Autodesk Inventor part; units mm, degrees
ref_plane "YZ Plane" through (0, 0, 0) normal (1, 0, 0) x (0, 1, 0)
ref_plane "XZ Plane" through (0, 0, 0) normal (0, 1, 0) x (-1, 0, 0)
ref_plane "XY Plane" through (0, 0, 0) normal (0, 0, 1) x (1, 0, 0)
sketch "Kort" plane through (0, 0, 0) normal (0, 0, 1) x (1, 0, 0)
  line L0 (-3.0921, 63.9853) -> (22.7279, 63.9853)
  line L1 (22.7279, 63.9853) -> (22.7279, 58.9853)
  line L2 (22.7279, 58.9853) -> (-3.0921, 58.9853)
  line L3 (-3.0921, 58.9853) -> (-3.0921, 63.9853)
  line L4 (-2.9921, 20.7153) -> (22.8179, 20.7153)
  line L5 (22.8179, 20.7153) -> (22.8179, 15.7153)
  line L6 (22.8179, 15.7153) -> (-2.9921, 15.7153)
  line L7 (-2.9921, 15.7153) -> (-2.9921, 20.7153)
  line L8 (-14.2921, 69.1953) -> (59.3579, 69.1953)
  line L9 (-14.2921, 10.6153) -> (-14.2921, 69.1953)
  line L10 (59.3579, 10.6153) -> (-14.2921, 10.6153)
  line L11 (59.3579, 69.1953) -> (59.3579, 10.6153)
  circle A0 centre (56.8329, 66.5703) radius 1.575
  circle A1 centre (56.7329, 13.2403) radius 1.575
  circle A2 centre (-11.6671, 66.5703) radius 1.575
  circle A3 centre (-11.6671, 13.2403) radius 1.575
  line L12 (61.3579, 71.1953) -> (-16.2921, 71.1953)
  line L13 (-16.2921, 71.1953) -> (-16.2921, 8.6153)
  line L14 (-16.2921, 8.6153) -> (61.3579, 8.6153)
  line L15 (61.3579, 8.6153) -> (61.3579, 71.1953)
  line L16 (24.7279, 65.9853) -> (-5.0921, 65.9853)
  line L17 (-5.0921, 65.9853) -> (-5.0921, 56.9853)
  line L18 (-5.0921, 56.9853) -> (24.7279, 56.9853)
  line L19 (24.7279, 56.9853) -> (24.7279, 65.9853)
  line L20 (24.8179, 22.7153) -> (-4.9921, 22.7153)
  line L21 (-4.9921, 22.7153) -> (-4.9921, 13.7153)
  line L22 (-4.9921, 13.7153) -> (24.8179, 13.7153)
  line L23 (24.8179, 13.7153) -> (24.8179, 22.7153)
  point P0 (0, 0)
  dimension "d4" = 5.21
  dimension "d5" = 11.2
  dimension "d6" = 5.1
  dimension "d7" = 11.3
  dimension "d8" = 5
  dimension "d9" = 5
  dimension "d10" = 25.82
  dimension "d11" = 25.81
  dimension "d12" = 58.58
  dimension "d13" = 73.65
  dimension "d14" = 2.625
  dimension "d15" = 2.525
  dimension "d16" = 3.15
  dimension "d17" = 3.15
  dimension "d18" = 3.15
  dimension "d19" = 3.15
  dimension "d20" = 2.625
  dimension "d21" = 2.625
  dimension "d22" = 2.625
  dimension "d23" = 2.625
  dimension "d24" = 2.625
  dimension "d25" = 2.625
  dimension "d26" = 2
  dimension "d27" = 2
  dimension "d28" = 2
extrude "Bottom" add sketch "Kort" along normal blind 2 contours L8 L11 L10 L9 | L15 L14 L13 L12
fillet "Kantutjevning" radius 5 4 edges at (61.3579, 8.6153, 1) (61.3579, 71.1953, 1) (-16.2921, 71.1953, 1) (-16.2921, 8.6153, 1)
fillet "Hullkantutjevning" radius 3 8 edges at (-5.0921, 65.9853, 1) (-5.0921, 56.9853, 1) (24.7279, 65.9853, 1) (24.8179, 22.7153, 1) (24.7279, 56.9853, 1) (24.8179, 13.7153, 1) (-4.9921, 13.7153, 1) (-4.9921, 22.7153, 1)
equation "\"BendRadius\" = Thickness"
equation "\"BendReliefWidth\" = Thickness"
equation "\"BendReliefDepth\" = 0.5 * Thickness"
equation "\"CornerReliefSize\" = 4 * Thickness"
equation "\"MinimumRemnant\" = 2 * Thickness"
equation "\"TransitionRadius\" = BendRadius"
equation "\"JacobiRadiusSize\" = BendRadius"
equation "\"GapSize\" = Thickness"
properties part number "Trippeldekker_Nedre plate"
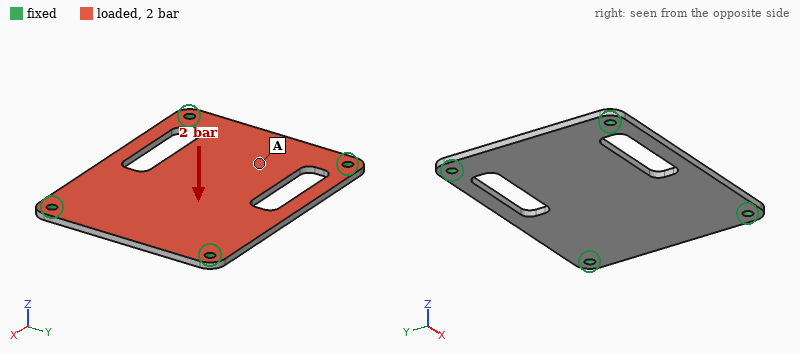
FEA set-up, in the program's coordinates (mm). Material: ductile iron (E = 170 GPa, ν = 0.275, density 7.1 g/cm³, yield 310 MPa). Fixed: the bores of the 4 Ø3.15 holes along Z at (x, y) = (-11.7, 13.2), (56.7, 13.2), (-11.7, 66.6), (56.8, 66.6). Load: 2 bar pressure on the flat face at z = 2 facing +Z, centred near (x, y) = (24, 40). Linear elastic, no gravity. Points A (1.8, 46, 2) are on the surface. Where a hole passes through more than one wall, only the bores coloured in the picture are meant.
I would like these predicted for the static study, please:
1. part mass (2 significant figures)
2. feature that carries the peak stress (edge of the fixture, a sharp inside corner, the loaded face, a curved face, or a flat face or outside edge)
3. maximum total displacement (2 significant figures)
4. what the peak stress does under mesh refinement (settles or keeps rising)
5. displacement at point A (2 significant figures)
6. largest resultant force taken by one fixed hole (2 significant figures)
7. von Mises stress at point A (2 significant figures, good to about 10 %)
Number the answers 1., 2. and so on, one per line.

1. 61 g
2. edge of the fixture
3. 0.19 mm
4. keeps rising
5. 0.13 mm
6. 230 N
7. 41 MPa
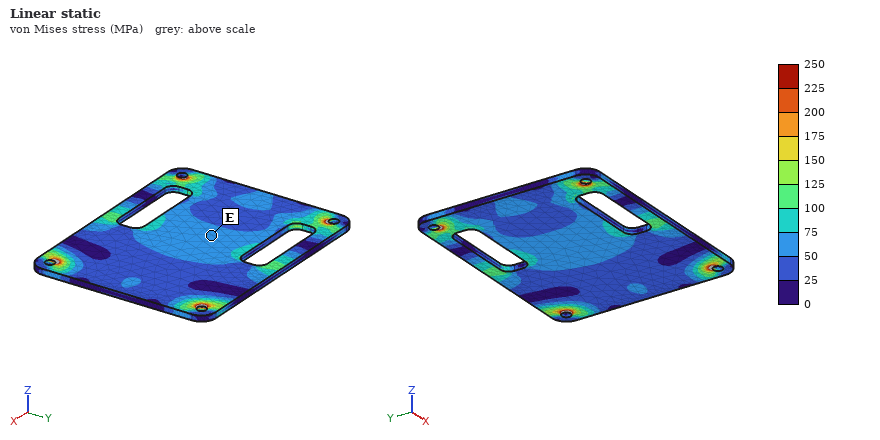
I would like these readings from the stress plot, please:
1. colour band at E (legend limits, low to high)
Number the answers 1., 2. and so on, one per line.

1. 50 to 75 MPa
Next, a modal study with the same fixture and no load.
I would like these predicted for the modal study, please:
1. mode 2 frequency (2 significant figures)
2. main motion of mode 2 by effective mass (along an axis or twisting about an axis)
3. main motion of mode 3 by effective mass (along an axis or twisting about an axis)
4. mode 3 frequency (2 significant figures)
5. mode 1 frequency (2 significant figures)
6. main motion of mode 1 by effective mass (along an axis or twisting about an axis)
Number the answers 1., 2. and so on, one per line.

1. 2700 Hz
2. twisting about X
3. twisting about Y
4. 3300 Hz
5. 1600 Hz
6. along Z
